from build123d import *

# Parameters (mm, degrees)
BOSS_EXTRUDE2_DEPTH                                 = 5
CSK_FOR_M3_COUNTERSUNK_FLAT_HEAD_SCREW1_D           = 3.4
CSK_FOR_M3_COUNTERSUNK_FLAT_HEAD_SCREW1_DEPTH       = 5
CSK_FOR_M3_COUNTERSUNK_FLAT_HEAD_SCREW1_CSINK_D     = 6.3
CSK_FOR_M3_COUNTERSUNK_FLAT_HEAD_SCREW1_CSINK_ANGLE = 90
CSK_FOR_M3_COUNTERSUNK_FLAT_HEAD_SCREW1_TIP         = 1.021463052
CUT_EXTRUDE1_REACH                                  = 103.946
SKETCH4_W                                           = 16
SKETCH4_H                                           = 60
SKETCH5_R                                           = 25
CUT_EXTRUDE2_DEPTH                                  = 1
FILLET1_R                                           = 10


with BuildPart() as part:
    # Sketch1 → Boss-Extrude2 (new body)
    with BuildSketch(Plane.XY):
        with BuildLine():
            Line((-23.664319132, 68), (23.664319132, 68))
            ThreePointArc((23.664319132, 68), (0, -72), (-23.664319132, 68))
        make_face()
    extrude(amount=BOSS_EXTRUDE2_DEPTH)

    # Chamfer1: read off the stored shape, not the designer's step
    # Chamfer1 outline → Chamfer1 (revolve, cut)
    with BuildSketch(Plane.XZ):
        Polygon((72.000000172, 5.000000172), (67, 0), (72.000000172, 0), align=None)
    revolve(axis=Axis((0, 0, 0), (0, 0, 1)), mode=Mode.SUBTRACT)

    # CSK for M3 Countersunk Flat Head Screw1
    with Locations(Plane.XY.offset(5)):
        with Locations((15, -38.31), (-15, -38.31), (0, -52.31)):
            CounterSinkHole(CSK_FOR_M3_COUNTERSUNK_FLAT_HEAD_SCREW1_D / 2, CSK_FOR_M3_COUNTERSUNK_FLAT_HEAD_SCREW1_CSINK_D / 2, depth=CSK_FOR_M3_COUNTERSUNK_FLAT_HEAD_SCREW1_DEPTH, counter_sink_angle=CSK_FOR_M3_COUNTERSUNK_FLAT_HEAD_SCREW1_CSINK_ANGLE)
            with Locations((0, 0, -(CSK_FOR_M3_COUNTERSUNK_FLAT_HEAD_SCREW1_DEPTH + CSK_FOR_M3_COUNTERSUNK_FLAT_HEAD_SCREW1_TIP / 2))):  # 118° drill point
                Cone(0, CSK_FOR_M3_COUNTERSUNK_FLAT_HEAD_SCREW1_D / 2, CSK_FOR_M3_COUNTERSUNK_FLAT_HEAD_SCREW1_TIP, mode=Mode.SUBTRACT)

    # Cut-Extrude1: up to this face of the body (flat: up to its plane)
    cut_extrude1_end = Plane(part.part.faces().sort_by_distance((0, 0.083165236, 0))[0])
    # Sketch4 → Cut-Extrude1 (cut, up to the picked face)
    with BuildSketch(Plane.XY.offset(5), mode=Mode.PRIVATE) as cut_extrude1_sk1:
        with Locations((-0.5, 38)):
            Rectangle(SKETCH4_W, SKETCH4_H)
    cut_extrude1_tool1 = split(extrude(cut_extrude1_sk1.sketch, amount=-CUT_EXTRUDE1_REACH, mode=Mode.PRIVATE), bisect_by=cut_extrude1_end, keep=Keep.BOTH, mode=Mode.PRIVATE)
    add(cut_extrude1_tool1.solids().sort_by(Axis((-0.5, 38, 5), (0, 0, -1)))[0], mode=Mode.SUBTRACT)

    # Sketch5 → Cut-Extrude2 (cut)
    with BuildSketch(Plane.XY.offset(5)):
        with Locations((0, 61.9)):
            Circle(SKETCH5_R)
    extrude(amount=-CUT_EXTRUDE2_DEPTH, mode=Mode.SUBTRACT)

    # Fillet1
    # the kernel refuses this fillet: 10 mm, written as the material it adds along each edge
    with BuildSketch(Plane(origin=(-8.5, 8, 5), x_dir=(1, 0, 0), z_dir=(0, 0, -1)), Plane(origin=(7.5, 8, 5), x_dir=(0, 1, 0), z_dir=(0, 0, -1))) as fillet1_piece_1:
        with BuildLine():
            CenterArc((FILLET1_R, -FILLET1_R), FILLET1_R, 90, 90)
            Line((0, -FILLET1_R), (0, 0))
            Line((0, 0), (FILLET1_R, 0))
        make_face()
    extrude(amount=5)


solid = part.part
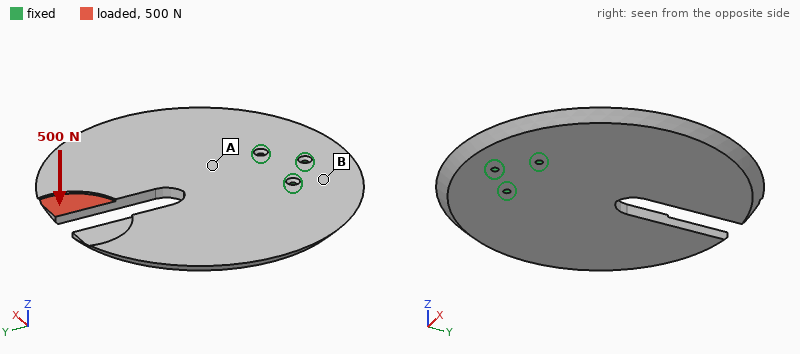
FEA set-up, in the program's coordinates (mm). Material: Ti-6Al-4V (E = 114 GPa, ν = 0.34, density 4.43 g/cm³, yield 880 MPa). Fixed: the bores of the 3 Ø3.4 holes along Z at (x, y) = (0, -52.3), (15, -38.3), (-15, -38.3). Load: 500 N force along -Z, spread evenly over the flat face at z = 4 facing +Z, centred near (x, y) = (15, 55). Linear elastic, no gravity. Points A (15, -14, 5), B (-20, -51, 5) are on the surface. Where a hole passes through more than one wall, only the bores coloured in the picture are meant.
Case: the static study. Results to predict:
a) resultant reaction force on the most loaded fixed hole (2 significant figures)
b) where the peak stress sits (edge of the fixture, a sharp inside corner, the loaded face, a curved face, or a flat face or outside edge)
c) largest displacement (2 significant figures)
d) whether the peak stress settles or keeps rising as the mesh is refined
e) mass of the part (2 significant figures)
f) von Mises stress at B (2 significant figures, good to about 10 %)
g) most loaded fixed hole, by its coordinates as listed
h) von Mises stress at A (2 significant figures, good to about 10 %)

1.3 kN
edge of the fixture
2.2 mm
keeps rising
310 g
34 MPa
(0, -52.3)
89 MPa
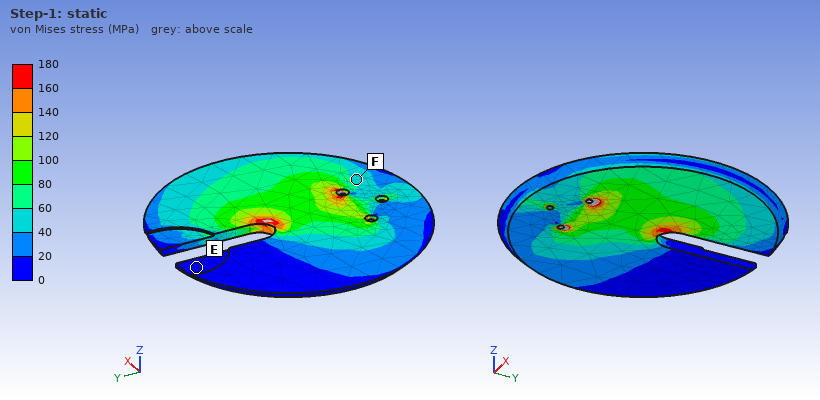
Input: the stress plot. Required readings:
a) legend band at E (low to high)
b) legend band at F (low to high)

0 to 20 MPa
40 to 60 MPa
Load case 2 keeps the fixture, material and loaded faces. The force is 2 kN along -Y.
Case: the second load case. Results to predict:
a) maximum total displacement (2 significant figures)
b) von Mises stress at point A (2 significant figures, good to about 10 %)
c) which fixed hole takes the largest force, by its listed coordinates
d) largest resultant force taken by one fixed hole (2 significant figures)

0.27 mm
19 MPa
(15, -38.3)
1.6 kN
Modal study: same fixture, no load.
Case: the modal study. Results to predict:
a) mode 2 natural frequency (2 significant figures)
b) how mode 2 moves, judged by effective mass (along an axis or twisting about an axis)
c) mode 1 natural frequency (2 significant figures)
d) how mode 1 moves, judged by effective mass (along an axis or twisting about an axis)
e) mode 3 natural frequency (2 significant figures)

540 Hz
twisting about Y
390 Hz
along Z
1200 Hz
